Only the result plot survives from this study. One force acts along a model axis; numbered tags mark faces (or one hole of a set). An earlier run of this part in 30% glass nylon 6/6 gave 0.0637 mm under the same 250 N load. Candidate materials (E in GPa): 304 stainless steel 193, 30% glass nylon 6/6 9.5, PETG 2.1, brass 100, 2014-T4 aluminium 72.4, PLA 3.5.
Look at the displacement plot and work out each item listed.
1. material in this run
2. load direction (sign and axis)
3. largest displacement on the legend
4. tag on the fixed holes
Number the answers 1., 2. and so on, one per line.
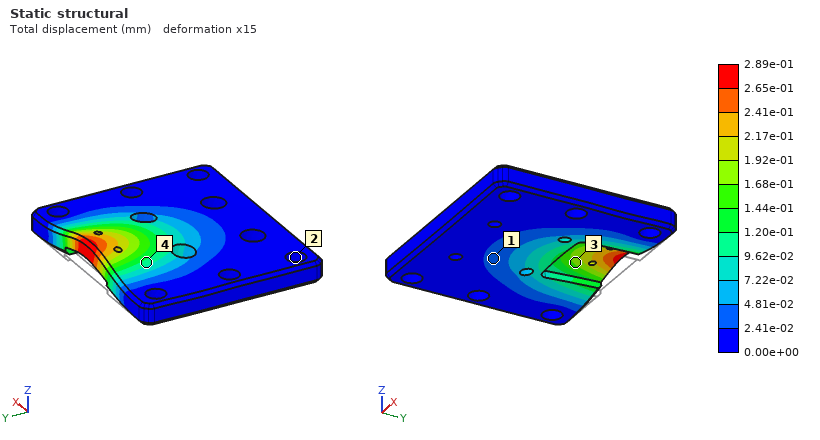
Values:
1. PETG
2. +Z
3. 2.89e-01 mm
4. 2
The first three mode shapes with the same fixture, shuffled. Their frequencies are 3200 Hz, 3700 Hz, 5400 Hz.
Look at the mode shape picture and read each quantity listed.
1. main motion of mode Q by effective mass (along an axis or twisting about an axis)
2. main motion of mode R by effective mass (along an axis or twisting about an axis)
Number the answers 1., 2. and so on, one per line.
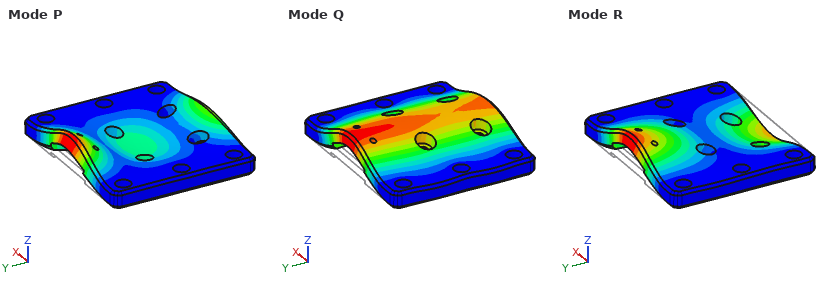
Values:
1. along Z
2. twisting about X
